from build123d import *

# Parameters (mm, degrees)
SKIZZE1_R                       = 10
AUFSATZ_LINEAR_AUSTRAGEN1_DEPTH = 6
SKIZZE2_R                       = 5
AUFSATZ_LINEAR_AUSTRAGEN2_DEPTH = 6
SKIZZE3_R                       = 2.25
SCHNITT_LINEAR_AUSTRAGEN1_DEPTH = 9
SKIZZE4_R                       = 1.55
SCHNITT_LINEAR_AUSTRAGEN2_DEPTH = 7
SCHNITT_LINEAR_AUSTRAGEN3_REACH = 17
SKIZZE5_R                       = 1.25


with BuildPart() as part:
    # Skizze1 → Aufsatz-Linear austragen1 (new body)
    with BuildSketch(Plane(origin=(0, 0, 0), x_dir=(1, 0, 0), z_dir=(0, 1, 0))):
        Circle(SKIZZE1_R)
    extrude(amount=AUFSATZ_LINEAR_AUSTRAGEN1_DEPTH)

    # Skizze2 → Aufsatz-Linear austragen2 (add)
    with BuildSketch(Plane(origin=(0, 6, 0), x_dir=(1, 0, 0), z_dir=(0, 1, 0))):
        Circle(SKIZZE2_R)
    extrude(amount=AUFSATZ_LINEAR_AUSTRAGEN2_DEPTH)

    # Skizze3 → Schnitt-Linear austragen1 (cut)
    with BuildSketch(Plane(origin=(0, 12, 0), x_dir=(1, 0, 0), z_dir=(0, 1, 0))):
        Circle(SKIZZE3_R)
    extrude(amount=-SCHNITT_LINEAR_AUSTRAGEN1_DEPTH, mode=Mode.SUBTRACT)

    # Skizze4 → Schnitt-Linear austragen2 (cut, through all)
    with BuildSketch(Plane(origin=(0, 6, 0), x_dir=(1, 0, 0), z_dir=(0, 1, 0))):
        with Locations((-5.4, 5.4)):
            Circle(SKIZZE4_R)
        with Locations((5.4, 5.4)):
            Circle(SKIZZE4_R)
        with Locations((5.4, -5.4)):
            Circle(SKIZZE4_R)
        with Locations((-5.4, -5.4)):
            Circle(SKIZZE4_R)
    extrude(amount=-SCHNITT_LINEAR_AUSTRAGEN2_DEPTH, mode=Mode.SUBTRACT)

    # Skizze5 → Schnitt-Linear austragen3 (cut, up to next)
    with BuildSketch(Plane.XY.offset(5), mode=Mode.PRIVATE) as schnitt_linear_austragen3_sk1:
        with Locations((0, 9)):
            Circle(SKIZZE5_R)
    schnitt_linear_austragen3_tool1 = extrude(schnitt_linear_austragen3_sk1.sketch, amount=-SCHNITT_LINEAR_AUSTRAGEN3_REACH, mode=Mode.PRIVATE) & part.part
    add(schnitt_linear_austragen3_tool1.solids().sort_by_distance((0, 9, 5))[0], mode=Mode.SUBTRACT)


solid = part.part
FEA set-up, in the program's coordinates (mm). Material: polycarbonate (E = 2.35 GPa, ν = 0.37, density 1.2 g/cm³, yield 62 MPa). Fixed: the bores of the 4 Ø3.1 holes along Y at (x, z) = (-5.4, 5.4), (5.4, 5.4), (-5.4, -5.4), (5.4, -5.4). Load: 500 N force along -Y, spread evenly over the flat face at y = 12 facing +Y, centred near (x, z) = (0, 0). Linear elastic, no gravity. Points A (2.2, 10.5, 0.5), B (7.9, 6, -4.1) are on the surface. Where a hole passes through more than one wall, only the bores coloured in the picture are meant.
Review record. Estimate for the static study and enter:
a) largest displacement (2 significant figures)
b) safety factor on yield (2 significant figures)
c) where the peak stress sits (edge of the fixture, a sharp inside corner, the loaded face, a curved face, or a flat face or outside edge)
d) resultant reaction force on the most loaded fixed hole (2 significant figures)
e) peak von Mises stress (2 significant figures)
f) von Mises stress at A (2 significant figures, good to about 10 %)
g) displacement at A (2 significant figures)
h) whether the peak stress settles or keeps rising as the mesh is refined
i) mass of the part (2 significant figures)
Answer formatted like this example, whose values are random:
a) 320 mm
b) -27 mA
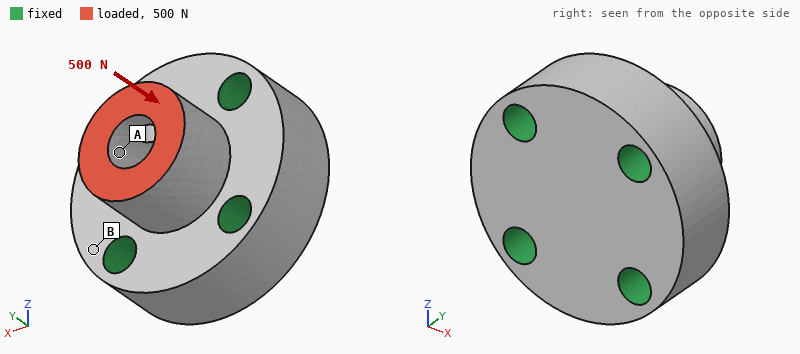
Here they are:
a) 54 µm
b) 2.0
c) a curved face
d) 130 N
e) 31 MPa
f) 8.8 MPa
g) 29 µm
h) settles
i) 2.4 g
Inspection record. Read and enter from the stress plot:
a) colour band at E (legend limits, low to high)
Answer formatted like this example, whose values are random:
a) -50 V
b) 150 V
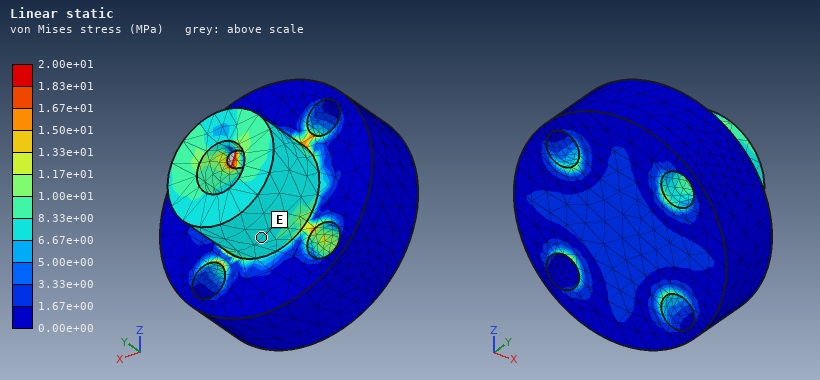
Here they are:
a) 6.67e+00 to 8.33e+00 MPa
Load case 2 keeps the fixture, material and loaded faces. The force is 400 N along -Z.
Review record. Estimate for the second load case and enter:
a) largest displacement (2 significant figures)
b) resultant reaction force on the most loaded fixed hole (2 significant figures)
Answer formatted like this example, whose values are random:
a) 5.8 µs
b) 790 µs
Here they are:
a) 0.19 mm
b) 190 N
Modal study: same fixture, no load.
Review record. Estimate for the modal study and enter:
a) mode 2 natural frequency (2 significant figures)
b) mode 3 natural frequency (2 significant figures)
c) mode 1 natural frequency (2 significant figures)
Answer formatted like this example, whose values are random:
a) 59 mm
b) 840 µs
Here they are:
a) 20 kHz
b) 28 kHz
c) 19 kHz
